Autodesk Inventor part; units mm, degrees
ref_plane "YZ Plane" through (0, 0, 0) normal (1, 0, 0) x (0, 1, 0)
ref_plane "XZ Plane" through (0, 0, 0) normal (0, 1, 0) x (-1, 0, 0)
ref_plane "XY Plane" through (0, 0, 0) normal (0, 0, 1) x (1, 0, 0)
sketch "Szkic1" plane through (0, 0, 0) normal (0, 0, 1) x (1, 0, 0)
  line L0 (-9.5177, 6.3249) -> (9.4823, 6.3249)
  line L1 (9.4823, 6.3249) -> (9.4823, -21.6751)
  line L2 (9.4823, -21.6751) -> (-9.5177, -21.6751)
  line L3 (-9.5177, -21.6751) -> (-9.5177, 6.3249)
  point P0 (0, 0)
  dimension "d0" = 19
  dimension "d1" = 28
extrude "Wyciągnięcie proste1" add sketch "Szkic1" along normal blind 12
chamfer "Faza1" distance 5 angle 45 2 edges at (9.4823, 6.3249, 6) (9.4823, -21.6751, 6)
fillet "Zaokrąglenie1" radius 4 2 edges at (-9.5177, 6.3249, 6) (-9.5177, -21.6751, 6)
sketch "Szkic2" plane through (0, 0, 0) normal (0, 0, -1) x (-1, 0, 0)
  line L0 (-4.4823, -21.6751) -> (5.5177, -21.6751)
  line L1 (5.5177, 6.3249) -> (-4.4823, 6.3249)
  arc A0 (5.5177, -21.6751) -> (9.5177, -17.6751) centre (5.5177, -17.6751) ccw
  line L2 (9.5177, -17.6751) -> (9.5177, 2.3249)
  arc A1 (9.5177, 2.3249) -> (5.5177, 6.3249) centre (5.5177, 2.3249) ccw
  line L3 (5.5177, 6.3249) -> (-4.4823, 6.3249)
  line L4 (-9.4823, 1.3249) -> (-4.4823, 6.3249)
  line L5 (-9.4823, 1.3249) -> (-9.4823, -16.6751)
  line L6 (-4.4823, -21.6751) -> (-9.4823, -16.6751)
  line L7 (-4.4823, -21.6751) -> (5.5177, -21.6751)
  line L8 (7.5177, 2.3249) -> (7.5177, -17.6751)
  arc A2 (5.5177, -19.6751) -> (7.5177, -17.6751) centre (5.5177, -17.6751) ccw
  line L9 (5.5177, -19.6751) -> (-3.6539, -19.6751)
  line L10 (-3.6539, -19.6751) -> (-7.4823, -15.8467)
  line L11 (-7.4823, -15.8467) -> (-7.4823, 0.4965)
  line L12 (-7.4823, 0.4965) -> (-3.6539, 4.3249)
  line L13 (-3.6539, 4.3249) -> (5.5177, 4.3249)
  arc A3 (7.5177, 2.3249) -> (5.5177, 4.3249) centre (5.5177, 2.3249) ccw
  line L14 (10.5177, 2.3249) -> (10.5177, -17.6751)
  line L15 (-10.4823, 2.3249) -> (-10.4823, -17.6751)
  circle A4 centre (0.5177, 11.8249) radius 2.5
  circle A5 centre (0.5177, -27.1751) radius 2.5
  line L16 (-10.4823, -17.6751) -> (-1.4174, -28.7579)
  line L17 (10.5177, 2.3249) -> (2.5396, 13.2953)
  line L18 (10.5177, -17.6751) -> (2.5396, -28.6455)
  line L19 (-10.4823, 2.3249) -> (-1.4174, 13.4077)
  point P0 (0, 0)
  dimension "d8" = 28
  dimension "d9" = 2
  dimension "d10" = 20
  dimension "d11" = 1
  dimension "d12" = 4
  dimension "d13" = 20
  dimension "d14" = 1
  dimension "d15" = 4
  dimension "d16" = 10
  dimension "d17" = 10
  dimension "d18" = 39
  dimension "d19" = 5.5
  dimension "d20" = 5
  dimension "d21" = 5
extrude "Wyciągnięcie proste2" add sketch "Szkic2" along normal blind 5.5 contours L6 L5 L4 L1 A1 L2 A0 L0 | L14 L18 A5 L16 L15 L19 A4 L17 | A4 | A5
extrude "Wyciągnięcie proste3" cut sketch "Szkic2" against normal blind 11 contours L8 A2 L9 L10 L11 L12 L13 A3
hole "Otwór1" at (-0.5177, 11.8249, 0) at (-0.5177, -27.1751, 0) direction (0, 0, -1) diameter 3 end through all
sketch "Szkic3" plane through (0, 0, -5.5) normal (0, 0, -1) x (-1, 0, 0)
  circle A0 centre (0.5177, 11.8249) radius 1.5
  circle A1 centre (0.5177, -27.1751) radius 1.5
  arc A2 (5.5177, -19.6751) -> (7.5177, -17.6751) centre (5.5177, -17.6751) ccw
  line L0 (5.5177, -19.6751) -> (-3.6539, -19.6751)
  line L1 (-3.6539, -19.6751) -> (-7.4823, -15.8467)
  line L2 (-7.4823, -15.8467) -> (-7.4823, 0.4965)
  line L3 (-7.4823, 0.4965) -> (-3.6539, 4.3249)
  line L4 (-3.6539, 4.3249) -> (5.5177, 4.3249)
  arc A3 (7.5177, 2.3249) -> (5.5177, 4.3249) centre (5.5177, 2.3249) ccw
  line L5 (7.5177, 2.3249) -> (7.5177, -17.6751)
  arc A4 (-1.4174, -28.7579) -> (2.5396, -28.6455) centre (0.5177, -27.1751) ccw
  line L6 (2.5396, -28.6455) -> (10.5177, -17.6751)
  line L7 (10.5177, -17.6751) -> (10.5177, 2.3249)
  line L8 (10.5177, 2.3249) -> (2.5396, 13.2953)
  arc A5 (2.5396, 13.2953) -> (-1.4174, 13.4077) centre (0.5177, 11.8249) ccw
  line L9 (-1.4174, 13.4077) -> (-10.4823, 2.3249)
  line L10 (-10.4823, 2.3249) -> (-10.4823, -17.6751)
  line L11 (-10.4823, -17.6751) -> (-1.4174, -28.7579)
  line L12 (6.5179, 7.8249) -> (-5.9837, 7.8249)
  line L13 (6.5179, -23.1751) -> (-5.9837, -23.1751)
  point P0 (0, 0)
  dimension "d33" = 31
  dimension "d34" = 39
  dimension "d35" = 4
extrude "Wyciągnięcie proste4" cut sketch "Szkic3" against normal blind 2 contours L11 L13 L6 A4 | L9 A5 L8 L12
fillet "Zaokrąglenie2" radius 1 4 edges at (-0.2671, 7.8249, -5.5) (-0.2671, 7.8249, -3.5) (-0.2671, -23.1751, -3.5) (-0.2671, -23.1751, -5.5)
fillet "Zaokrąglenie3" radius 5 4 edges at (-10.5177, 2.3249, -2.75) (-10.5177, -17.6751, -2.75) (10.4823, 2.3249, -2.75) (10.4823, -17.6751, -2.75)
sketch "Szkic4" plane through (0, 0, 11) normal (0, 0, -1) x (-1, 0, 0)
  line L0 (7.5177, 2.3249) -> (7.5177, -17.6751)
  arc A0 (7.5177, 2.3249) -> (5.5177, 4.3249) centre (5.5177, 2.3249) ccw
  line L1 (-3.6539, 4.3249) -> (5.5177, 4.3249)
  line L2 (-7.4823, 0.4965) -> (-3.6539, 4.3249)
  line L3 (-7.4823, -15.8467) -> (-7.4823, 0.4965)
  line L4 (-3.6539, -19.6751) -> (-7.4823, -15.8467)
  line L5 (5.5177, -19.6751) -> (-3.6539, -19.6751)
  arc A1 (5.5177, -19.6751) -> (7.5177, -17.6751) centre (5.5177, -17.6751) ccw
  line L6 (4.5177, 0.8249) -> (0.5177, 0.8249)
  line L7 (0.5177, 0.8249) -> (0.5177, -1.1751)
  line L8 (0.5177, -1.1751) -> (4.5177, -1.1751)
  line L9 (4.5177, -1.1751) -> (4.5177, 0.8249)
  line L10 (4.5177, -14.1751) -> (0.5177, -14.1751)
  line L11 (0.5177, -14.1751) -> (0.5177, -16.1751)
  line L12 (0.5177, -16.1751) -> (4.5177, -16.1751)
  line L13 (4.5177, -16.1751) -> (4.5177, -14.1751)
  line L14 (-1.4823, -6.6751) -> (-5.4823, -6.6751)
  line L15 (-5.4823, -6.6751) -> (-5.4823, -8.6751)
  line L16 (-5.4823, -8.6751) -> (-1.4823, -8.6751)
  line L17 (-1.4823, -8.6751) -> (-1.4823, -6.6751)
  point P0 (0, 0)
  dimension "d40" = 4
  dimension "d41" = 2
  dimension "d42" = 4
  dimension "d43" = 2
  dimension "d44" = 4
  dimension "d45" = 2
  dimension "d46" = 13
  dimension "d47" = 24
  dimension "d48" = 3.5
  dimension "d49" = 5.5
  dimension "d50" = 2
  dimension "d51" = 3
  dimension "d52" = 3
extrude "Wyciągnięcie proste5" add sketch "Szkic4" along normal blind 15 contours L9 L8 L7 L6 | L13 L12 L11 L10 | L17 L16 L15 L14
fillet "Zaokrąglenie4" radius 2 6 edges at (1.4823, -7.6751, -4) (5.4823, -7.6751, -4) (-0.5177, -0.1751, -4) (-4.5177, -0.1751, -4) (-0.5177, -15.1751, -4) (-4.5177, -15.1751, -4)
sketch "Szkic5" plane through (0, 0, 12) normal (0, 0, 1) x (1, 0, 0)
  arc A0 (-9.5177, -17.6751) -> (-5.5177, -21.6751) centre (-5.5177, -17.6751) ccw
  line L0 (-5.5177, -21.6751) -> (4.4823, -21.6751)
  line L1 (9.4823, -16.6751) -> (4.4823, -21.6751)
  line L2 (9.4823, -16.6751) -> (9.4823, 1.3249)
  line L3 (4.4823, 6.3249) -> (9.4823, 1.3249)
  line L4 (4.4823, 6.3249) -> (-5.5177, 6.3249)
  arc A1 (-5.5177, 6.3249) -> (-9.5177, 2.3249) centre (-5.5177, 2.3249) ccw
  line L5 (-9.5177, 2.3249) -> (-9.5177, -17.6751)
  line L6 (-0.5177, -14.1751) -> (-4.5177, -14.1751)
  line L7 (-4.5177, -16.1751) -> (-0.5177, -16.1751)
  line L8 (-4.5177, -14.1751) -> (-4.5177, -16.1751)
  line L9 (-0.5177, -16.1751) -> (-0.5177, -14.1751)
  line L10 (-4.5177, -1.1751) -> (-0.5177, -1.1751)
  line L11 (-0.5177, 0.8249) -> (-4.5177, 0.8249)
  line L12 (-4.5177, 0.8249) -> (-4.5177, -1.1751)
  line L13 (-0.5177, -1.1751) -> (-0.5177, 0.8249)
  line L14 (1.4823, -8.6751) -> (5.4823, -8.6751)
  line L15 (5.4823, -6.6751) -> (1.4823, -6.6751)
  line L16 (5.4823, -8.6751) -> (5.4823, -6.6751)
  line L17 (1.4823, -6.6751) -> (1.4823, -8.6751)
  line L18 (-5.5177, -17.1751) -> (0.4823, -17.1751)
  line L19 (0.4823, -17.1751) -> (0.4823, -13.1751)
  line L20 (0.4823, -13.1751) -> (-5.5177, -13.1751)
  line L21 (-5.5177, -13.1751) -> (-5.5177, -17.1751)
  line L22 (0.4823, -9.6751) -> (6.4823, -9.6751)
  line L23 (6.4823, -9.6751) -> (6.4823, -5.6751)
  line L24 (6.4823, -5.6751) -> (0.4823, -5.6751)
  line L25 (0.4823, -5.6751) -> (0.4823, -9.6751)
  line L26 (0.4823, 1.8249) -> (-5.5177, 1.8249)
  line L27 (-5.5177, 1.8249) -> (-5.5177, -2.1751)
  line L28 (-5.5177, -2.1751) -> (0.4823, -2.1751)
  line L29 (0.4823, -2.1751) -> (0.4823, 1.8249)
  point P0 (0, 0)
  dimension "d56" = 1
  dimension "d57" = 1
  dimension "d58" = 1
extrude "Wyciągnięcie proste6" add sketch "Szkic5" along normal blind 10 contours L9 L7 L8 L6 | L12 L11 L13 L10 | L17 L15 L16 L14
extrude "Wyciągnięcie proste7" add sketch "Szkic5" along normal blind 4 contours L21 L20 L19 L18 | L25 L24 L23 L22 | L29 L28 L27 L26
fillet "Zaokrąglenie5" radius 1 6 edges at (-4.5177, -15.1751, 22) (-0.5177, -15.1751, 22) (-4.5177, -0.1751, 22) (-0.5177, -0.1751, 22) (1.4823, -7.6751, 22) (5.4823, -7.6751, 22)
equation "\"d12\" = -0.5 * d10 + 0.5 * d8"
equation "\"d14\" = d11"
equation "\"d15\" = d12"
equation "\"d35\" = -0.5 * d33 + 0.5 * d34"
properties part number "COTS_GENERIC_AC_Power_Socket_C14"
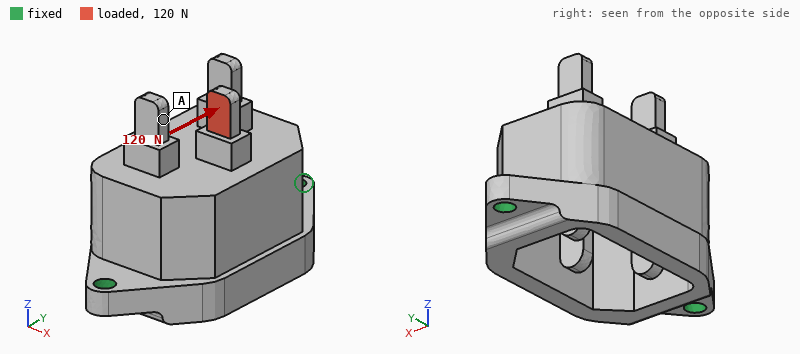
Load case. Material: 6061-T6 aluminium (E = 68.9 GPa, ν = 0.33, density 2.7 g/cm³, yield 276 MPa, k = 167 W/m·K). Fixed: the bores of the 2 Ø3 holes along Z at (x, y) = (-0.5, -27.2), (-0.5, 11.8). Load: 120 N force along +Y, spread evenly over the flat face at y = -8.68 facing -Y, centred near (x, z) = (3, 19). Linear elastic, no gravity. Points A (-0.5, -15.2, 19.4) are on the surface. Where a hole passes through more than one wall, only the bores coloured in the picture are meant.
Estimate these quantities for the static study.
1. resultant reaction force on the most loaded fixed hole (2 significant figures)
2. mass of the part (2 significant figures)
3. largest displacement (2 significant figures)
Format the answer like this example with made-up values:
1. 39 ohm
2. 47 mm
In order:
1. 98 N
2. 13 g
3. 78 µm
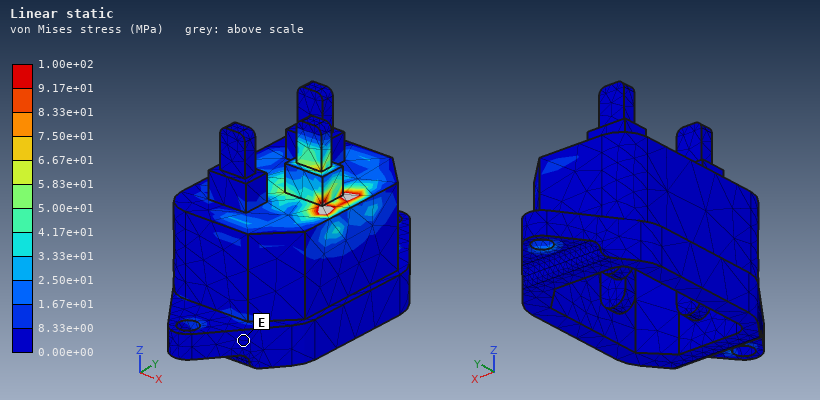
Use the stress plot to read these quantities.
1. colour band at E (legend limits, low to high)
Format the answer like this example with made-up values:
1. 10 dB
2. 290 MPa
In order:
1. 0.00e+00 to 8.33e+00 MPa
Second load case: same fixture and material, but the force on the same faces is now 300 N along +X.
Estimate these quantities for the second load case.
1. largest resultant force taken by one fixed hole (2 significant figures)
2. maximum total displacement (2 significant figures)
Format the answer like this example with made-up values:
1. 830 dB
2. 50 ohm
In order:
1. 160 N
2. 0.26 mm
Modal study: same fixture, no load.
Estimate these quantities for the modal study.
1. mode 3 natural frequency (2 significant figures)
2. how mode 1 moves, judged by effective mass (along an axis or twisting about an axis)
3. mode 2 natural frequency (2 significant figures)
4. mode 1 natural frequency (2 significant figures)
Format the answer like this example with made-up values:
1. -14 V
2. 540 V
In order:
1. 6200 Hz
2. along X
3. 6100 Hz
4. 4700 Hz
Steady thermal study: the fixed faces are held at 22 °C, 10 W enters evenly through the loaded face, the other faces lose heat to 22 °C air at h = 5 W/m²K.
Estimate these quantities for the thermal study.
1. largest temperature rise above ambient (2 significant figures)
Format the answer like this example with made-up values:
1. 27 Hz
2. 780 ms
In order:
1. 60 K
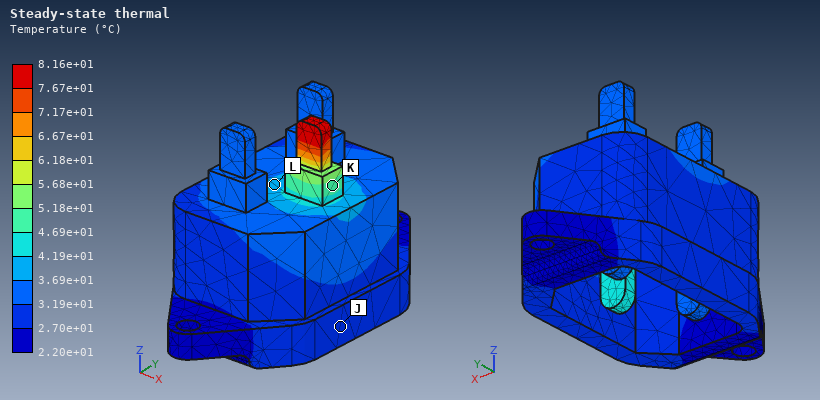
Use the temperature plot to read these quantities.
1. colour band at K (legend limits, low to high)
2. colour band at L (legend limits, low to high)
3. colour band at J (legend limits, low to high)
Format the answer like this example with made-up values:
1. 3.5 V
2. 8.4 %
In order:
1. 4.69e+01 to 5.18e+01 °C
2. 3.69e+01 to 4.19e+01 °C
3. 2.70e+01 to 3.19e+01 °C
